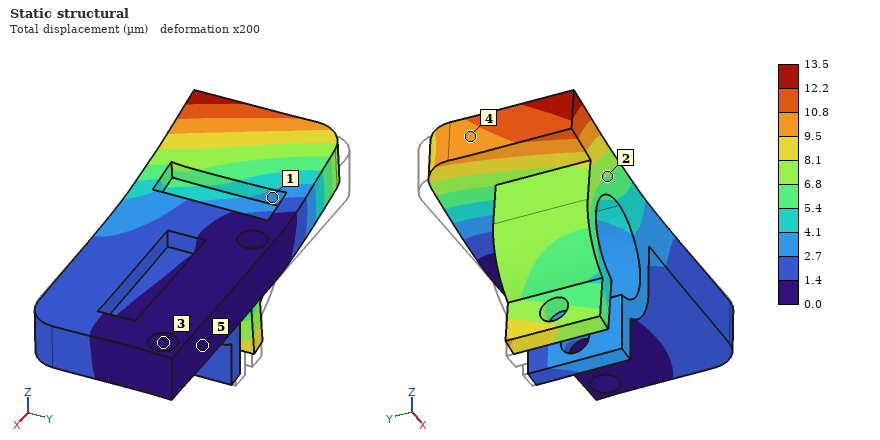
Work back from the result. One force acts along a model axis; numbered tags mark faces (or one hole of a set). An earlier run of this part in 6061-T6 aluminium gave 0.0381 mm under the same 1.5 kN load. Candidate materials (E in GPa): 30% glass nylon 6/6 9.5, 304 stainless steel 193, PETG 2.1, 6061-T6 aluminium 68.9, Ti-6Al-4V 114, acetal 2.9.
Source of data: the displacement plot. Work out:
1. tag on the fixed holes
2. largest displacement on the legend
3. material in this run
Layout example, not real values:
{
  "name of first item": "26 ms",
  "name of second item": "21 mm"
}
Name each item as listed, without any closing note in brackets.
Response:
{
  "tag on the fixed holes": "3",
  "largest displacement on the legend": "13.5 µm",
  "material in this run": "304 stainless steel"
}
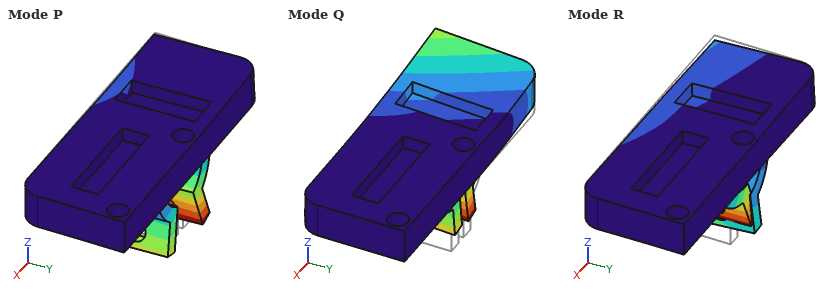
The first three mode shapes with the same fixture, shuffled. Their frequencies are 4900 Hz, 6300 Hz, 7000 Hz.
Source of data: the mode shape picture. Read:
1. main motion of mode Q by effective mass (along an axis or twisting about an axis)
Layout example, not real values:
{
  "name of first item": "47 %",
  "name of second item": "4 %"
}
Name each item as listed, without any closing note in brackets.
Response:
{
  "main motion of mode Q by effective mass": "along Z"
}
